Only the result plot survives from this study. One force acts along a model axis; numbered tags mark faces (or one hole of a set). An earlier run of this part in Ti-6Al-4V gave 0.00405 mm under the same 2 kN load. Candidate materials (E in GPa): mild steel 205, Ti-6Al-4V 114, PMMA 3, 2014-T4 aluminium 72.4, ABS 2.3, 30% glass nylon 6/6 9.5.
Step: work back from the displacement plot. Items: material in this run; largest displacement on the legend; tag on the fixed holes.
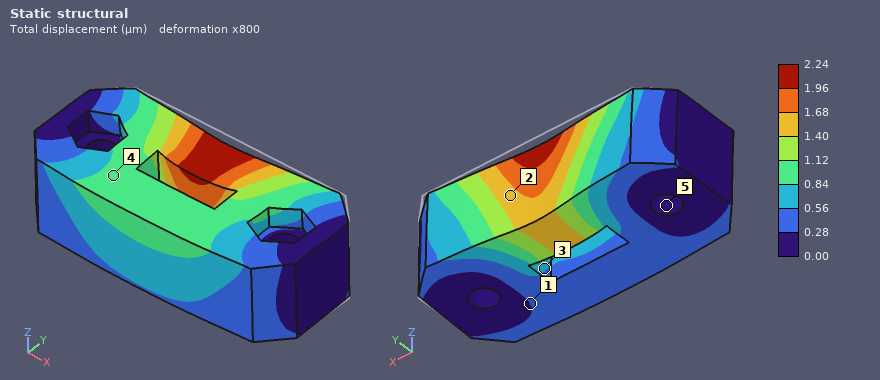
mild steel
2.24 µm
5
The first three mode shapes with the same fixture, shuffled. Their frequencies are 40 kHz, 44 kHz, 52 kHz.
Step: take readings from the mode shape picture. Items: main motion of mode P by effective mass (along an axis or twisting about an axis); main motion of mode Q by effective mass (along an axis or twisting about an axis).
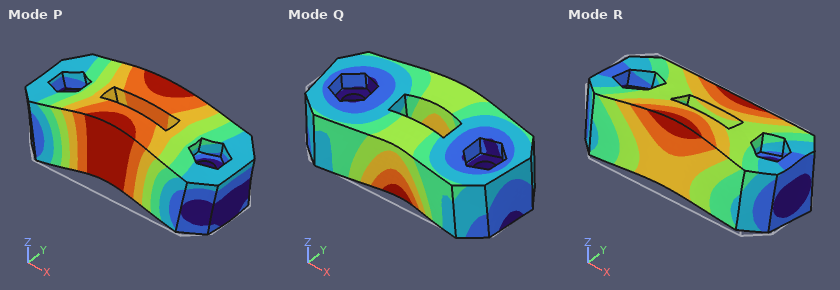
along Z
along Y
